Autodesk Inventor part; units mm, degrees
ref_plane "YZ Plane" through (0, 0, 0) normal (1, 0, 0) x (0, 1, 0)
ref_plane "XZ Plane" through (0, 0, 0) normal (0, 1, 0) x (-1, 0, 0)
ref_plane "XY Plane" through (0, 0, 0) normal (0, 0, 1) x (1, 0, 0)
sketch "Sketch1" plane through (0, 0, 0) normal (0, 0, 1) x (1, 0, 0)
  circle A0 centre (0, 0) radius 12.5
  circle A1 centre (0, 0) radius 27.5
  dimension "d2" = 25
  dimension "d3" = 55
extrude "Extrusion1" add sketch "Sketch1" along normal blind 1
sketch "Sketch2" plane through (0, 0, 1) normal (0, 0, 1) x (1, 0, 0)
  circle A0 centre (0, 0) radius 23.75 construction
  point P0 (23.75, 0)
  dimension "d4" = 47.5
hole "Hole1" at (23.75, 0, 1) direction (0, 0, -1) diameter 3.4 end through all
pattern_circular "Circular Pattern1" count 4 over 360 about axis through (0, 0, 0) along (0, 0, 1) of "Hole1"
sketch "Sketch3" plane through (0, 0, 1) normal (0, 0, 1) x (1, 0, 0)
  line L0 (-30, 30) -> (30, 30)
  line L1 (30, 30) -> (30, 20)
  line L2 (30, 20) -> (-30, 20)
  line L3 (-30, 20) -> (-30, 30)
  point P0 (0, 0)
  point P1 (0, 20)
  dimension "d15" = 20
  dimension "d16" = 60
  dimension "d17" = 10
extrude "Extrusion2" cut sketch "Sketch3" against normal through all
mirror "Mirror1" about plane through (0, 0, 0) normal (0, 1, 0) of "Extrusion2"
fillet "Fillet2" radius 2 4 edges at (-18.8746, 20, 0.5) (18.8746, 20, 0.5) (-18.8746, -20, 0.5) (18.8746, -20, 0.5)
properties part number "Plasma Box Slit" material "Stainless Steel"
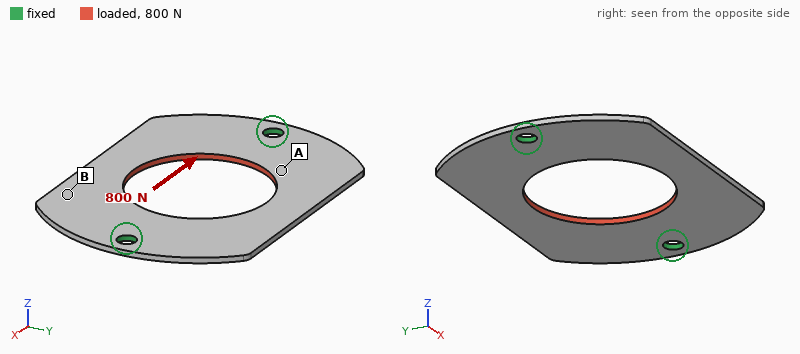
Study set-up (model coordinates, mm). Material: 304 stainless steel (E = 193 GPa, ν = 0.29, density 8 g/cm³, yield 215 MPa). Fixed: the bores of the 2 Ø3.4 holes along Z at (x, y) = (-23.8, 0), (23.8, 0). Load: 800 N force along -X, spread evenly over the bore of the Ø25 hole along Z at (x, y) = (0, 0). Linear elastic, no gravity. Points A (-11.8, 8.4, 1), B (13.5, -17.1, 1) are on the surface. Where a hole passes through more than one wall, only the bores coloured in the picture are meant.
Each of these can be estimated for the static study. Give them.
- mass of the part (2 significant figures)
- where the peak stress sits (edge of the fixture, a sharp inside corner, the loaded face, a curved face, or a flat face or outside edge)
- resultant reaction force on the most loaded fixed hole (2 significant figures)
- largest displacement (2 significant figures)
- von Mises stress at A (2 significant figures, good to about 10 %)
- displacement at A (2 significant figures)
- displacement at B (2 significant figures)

12 g
edge of the fixture
400 N
4.2 µm
22 MPa
2.9 µm
3.5 µm
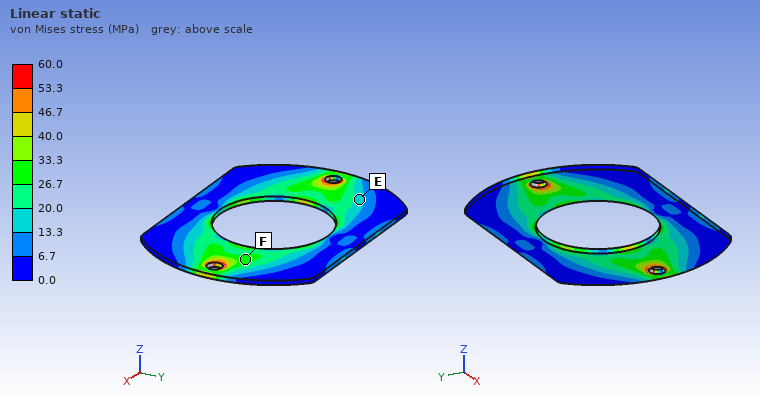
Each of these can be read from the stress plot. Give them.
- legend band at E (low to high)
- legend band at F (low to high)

13.3 to 20.0 MPa
26.7 to 33.3 MPa
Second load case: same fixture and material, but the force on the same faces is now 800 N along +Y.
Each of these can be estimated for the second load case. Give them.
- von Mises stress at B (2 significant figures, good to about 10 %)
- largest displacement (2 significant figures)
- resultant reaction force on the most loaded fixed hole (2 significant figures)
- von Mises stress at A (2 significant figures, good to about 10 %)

13 MPa
5.7 µm
400 N
25 MPa
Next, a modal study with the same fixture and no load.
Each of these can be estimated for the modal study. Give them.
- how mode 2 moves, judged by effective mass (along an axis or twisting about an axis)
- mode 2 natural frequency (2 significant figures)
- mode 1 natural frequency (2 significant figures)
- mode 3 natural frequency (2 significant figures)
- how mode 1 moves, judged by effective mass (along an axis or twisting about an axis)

along Z
1500 Hz
1300 Hz
2800 Hz
twisting about X
